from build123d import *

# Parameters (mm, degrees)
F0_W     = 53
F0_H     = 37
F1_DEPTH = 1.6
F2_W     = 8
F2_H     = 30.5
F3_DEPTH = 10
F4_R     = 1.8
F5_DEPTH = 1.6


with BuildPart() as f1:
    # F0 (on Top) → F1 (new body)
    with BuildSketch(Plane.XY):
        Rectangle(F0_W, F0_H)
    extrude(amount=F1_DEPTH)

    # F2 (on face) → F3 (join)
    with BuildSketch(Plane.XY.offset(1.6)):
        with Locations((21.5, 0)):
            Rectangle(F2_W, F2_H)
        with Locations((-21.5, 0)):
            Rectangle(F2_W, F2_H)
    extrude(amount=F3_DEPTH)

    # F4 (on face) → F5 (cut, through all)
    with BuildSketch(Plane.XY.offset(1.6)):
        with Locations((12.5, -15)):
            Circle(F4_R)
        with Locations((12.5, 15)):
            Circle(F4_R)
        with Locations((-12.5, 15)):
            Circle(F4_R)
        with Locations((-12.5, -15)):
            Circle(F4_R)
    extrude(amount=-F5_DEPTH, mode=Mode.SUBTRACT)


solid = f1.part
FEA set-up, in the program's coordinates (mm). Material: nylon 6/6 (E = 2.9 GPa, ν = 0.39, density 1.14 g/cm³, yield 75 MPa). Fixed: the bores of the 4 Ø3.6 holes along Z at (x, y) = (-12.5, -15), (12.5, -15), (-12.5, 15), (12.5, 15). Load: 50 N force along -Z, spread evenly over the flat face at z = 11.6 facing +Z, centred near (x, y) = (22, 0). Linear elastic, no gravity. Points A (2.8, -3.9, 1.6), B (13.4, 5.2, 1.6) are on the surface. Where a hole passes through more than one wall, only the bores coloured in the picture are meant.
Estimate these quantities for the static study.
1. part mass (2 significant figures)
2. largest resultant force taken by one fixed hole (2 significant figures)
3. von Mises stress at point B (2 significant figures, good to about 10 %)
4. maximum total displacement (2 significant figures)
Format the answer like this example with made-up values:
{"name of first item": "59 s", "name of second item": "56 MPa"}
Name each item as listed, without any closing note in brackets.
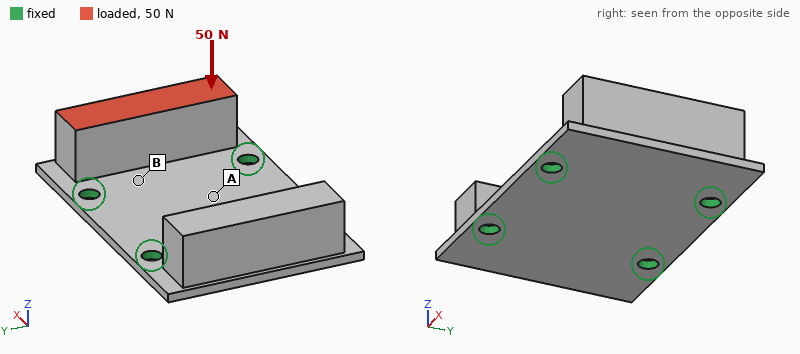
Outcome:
{"part mass": "9.1 g", "largest resultant force taken by one fixed hole": "27 N", "von Mises stress at point B": "9.2 MPa", "maximum total displacement": "0.61 mm"}
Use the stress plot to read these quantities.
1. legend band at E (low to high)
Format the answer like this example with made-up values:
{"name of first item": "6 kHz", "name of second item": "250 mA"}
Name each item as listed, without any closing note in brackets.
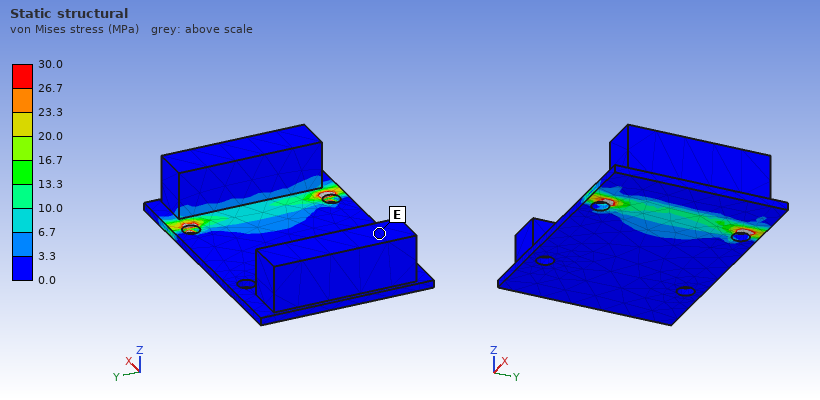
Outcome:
{"legend band at E": "0.0 to 3.3 MPa"}
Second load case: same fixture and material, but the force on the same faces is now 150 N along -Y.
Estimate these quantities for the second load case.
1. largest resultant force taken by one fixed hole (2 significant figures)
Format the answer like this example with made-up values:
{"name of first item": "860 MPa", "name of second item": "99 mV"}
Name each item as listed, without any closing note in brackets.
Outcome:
{"largest resultant force taken by one fixed hole": "100 N"}
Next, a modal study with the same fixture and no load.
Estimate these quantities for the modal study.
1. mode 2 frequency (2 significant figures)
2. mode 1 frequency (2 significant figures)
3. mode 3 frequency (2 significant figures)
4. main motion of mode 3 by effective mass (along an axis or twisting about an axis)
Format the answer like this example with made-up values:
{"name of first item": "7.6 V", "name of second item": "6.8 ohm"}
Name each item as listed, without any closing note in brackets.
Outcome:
{"mode 2 frequency": "840 Hz", "mode 1 frequency": "820 Hz", "mode 3 frequency": "3200 Hz", "main motion of mode 3 by effective mass": "along Z"}
